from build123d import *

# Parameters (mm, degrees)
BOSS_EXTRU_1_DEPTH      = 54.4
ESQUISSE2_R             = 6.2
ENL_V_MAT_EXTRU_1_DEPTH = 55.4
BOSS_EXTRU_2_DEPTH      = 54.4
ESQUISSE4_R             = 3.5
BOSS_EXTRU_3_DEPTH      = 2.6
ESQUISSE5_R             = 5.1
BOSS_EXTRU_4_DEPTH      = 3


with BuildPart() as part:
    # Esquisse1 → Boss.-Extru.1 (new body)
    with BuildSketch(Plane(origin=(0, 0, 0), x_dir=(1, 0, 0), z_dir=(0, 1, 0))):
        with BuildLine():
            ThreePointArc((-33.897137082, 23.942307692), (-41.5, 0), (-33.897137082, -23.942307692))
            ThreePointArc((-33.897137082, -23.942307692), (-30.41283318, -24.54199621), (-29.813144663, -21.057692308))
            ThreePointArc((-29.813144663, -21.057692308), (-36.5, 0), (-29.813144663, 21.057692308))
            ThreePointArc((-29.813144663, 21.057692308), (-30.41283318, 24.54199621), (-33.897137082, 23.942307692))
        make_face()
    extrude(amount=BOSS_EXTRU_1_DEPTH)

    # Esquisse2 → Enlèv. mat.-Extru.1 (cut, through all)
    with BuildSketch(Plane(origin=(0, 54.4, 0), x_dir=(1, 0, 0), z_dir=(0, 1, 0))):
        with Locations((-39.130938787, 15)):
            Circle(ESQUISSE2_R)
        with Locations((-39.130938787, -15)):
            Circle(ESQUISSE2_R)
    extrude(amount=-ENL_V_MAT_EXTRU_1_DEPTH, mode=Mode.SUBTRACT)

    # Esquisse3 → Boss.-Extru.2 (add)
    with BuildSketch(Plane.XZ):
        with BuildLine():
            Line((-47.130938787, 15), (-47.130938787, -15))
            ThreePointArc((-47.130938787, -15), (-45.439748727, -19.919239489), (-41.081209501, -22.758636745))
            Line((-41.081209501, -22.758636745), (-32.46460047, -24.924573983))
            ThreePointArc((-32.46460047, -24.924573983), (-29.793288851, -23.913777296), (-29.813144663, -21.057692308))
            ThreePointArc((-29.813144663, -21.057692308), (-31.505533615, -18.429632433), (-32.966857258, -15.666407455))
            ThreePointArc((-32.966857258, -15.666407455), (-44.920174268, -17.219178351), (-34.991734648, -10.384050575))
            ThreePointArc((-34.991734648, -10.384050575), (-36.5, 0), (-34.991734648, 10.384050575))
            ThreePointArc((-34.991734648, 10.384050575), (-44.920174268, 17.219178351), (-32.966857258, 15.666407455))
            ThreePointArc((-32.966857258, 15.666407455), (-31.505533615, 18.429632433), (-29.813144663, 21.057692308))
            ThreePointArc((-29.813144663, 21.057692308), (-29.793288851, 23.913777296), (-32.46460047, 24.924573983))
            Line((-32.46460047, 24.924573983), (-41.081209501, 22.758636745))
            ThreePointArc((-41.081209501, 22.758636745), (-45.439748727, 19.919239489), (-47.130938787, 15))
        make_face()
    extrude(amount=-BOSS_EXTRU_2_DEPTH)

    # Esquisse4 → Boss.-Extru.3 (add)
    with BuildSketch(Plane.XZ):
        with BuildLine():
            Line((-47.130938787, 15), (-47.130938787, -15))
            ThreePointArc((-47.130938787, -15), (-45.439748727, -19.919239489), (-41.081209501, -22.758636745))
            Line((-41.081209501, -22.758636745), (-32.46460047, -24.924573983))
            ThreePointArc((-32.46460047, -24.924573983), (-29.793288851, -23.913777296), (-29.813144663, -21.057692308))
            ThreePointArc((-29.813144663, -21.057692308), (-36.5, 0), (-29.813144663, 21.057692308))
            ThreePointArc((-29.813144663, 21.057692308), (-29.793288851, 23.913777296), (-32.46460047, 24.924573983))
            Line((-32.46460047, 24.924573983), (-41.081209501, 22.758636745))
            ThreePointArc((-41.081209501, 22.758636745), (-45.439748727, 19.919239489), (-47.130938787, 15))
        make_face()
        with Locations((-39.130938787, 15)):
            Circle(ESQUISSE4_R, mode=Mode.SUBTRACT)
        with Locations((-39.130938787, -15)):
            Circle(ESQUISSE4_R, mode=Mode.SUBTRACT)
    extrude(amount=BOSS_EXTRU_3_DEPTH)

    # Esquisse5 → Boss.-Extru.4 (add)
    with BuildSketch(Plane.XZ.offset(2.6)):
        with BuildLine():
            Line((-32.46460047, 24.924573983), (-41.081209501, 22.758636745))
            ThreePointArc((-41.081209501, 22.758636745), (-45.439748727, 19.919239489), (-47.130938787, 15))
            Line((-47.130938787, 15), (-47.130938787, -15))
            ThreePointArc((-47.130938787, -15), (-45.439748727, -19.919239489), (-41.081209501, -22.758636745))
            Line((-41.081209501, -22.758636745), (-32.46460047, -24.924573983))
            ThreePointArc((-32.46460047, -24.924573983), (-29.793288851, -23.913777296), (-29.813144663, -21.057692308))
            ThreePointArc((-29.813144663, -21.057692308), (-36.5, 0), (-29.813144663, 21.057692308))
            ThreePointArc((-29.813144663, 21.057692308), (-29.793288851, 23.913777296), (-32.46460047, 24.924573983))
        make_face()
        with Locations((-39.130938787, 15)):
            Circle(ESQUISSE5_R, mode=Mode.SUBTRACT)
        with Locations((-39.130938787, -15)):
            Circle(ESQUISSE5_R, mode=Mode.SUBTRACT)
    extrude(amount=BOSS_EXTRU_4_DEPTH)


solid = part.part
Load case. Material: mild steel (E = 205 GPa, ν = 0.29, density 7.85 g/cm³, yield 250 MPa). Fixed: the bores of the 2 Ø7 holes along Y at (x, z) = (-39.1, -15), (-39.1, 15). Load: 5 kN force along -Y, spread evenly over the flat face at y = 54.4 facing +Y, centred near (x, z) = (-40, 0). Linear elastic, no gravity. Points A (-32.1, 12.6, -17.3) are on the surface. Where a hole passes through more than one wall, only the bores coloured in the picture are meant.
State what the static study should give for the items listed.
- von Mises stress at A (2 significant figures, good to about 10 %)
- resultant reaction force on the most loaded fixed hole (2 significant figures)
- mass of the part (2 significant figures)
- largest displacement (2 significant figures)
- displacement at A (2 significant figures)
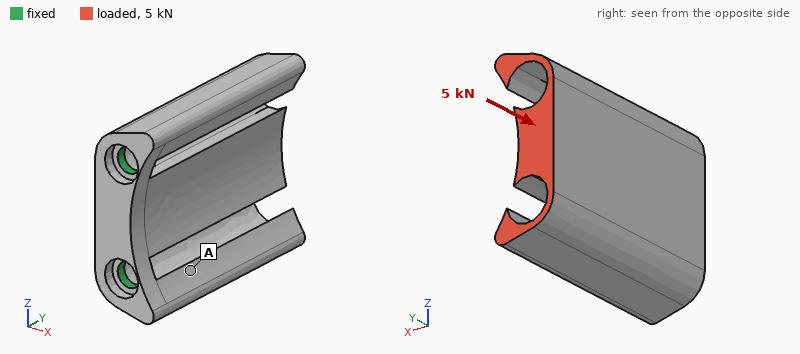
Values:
20 MPa
2.5 kN
180 g
7.5 µm
4.1 µm
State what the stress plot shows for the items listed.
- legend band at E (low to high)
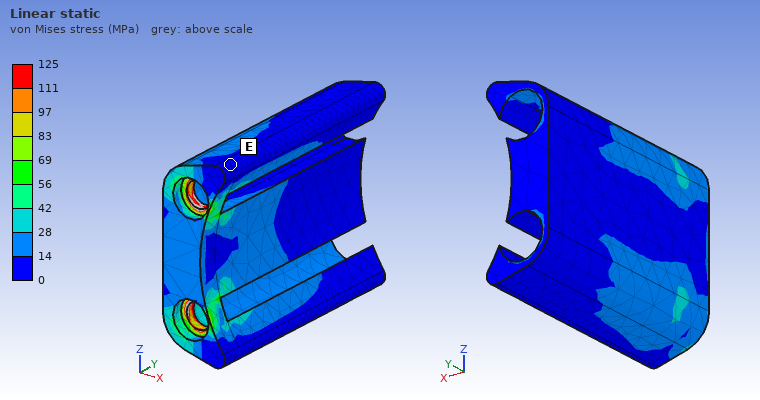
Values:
0 to 14 MPa
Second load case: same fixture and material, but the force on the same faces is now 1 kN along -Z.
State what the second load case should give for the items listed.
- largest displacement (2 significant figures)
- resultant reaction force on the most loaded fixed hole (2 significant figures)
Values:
79 µm
1.9 kN
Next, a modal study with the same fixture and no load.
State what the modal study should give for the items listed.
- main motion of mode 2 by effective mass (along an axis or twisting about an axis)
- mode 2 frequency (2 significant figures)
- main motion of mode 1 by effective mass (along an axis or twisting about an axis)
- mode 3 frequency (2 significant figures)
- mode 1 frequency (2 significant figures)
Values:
along Z
3200 Hz
along X
4000 Hz
1600 Hz
